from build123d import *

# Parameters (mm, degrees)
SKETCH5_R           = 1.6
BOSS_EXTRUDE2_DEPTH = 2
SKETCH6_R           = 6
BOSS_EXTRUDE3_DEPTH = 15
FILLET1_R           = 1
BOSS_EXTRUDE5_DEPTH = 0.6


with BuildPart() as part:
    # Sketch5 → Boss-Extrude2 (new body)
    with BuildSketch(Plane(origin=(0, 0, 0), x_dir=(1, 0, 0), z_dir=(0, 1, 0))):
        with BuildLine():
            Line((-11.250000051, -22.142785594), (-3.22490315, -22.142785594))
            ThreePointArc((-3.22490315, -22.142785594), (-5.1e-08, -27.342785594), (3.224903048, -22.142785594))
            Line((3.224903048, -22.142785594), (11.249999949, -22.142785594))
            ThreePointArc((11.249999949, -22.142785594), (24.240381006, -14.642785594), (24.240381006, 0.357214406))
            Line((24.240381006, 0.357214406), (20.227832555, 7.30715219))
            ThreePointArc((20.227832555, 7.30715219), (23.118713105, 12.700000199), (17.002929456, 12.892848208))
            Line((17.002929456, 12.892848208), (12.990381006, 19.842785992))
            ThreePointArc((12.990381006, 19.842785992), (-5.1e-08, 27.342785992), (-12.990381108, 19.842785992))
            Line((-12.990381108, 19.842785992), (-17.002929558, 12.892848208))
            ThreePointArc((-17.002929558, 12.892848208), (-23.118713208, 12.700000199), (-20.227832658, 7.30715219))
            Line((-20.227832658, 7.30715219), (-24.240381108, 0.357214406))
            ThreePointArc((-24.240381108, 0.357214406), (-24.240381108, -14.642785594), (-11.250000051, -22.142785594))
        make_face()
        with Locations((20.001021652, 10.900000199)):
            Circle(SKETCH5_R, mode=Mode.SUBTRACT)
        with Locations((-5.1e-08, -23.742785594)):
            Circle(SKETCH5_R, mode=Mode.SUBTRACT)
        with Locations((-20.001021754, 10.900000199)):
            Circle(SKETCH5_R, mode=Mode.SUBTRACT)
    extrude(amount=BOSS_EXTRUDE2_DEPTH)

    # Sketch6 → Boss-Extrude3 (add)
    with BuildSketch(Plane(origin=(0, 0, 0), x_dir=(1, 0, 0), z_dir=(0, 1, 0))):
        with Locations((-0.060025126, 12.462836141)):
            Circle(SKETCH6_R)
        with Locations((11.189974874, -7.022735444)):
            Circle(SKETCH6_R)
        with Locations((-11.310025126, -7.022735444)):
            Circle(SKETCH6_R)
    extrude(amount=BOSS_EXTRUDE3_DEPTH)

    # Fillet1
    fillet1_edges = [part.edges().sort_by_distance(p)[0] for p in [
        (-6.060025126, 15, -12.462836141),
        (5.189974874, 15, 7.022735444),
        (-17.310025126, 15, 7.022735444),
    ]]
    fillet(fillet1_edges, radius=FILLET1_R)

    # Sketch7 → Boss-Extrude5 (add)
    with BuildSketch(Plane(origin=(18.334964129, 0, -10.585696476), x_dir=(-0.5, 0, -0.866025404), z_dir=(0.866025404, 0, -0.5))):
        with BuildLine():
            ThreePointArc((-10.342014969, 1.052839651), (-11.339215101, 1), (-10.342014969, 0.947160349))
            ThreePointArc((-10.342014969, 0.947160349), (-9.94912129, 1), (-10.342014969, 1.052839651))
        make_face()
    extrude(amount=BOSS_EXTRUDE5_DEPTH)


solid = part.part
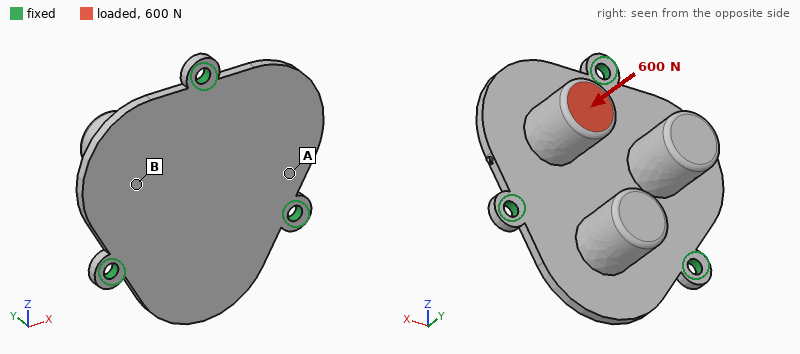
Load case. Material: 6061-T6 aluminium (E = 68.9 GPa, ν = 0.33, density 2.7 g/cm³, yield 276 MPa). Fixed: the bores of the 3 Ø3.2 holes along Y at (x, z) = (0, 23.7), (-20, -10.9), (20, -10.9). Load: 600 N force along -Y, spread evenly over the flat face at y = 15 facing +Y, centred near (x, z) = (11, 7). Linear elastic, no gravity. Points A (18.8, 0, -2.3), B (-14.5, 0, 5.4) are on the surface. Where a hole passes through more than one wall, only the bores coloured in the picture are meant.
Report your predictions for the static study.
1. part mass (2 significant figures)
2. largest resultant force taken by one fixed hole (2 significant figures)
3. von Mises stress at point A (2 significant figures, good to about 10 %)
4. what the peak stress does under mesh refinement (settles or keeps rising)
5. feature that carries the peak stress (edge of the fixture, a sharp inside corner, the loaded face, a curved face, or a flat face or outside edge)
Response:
23 g
320 N
51 MPa
keeps rising
edge of the fixture
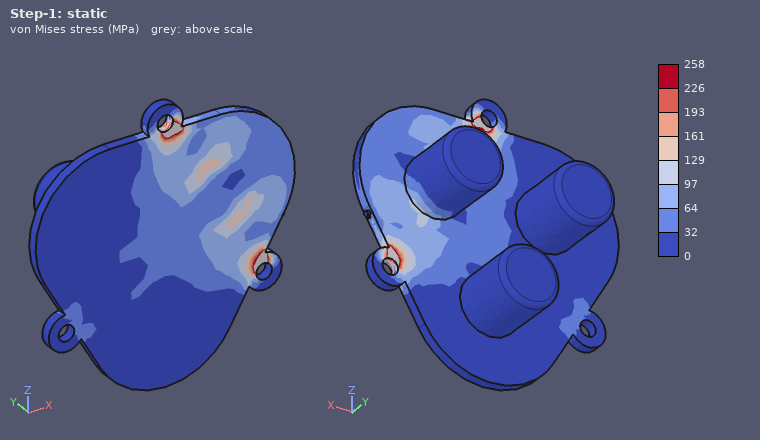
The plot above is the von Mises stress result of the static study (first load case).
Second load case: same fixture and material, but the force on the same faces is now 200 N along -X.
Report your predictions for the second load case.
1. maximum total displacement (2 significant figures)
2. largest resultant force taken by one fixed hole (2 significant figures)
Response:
0.15 mm
100 N
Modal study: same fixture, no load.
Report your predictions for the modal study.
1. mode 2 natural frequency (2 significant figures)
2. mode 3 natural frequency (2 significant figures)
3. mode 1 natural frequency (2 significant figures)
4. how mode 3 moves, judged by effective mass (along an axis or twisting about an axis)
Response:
3000 Hz
3600 Hz
3000 Hz
along Y
